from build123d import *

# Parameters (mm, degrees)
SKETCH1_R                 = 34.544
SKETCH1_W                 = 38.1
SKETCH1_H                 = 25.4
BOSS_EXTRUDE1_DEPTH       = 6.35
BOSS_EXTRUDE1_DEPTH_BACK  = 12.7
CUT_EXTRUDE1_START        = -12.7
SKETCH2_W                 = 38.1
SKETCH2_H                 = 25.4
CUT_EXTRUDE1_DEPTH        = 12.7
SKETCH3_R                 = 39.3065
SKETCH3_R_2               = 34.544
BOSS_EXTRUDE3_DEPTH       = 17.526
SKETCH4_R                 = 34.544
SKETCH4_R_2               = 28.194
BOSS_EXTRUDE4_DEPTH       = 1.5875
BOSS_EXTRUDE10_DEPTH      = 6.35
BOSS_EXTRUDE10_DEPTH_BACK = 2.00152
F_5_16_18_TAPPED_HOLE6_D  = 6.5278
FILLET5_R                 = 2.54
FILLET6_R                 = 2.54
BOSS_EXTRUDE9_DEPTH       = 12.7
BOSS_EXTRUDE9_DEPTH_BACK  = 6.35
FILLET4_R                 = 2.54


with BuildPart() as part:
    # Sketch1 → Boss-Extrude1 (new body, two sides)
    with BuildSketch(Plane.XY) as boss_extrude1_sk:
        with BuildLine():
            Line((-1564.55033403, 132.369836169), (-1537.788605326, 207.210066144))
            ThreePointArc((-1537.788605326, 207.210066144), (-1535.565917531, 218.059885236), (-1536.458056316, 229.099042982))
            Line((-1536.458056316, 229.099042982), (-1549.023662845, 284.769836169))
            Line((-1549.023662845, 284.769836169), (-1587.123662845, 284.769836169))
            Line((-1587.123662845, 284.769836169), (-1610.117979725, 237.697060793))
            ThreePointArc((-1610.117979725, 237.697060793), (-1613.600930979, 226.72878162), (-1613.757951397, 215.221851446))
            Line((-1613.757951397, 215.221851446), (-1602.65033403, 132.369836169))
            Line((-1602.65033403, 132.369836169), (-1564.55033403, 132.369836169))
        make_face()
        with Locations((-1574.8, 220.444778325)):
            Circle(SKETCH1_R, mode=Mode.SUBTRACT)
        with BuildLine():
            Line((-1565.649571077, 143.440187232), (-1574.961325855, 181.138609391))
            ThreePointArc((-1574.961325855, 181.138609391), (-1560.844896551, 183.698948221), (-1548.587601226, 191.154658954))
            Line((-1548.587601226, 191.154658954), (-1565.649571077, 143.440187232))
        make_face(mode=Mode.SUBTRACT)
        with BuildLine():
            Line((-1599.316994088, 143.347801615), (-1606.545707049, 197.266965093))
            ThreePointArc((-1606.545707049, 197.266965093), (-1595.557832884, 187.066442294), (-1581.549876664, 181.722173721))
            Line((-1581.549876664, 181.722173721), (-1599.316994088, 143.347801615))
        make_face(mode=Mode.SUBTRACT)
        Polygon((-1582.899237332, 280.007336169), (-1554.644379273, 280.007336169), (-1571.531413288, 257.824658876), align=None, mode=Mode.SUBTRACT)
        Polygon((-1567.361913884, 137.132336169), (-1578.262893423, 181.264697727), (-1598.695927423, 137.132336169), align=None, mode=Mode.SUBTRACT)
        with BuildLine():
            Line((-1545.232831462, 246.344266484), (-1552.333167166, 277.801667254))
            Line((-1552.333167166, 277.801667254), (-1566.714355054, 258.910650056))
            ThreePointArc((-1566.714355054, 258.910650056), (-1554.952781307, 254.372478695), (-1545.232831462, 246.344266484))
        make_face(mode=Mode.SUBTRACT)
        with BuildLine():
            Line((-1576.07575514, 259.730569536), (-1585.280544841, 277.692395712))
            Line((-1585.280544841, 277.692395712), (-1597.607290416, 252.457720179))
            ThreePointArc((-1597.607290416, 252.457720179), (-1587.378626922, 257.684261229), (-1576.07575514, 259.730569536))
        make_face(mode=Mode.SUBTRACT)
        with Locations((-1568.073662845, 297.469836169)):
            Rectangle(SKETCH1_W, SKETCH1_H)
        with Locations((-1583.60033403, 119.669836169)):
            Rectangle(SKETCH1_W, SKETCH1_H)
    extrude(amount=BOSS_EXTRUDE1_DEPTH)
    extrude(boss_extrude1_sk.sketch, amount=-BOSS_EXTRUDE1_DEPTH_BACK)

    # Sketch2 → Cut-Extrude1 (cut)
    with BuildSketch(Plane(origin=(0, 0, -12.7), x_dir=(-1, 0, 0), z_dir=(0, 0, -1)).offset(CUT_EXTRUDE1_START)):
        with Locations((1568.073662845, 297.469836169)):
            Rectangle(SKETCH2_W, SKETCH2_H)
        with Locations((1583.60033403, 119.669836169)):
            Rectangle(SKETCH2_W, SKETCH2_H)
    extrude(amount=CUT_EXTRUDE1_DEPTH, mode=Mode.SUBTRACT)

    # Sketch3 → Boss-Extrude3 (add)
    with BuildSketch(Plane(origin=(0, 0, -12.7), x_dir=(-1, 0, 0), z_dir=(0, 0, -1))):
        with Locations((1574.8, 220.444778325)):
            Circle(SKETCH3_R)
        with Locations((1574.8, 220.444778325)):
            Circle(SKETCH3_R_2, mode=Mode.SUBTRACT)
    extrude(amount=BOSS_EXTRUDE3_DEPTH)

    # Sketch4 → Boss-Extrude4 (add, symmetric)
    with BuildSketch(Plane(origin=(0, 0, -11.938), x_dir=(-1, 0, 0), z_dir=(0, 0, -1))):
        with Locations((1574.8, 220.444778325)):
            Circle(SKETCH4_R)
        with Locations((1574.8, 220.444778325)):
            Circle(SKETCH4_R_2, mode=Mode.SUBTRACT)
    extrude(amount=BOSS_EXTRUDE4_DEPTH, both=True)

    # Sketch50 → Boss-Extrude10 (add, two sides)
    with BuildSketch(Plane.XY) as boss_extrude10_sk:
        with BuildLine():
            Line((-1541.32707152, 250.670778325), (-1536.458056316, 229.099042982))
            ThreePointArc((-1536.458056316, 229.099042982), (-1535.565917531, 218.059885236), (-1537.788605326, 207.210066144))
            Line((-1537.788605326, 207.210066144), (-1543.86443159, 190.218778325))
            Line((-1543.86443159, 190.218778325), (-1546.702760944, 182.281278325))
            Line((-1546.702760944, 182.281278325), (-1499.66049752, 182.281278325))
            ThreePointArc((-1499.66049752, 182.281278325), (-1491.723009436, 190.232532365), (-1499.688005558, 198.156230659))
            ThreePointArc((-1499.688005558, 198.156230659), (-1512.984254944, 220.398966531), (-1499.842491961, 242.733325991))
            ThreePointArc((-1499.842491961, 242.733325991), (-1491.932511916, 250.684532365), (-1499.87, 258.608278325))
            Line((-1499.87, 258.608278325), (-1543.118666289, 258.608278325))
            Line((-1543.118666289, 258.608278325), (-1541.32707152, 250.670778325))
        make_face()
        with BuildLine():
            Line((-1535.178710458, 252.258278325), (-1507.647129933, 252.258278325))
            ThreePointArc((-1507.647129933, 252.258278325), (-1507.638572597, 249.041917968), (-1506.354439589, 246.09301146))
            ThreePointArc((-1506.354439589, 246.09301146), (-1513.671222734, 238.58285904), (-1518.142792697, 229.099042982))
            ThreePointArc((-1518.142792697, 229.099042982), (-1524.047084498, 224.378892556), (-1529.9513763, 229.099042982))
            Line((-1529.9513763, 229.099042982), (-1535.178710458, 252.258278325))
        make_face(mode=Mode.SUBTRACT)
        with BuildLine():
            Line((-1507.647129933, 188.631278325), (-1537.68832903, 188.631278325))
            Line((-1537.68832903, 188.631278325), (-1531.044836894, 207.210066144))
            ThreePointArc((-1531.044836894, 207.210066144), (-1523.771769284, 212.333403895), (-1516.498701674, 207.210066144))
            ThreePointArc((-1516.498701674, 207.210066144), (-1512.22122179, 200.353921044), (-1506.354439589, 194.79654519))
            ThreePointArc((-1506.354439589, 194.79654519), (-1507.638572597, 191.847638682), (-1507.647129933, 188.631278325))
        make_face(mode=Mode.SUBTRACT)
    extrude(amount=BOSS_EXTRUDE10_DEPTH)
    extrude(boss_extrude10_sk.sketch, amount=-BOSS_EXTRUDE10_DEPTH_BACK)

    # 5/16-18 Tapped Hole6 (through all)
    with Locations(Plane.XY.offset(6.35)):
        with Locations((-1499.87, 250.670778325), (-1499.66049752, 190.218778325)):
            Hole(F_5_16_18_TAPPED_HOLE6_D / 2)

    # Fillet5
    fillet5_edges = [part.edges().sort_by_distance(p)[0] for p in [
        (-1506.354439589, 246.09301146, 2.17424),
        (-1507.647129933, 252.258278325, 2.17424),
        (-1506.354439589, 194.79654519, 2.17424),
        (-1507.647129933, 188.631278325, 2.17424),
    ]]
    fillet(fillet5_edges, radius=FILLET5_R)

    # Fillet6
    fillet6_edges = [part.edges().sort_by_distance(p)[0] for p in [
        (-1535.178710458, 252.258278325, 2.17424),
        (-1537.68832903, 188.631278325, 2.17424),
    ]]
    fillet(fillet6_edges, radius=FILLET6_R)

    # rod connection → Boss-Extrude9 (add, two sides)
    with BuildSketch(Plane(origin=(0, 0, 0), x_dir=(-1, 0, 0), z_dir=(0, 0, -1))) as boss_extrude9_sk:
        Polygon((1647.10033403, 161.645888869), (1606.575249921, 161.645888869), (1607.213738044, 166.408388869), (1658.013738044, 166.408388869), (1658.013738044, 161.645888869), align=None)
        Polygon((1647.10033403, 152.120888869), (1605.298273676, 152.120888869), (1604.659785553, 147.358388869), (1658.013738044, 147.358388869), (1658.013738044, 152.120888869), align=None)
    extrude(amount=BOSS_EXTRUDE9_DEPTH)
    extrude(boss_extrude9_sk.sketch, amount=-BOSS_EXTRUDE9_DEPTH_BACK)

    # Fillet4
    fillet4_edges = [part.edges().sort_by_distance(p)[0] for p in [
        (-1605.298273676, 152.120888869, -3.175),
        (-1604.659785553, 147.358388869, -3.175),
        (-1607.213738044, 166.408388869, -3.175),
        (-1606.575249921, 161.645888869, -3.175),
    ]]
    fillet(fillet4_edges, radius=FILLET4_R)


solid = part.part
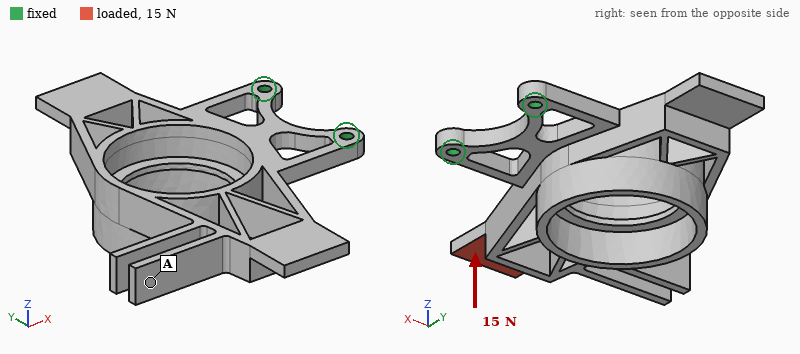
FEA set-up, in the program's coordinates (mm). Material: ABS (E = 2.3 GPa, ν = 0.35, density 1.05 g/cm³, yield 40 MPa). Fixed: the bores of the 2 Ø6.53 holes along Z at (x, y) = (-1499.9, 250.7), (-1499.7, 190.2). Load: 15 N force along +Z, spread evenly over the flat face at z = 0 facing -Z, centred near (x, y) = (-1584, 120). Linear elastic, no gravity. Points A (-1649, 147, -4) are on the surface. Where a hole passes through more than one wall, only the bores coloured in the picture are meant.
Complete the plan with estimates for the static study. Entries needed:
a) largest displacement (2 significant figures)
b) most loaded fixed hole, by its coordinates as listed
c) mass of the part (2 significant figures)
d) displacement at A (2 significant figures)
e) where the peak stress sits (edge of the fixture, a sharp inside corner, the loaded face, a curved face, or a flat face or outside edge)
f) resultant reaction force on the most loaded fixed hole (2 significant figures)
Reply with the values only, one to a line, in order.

2.9 mm
(-1499.7, 190.2)
120 g
2.7 mm
a curved face
31 N
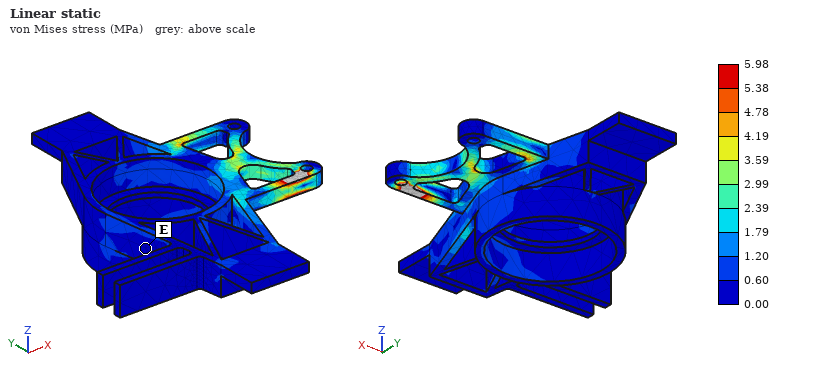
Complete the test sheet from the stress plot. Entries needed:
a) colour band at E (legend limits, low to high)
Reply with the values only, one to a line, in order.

0.00 to 0.60 MPa
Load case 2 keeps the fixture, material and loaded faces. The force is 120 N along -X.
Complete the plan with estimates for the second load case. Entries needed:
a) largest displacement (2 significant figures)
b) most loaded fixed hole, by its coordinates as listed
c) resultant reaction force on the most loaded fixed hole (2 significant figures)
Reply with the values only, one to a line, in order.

2.6 mm
(-1499.7, 190.2)
240 N
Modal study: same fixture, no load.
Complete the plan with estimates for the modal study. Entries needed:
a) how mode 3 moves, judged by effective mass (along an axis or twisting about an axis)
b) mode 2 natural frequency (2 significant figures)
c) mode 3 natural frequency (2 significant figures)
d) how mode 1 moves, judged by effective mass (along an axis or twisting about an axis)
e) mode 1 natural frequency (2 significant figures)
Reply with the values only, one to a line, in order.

along Y
140 Hz
200 Hz
along Z
55 Hz
